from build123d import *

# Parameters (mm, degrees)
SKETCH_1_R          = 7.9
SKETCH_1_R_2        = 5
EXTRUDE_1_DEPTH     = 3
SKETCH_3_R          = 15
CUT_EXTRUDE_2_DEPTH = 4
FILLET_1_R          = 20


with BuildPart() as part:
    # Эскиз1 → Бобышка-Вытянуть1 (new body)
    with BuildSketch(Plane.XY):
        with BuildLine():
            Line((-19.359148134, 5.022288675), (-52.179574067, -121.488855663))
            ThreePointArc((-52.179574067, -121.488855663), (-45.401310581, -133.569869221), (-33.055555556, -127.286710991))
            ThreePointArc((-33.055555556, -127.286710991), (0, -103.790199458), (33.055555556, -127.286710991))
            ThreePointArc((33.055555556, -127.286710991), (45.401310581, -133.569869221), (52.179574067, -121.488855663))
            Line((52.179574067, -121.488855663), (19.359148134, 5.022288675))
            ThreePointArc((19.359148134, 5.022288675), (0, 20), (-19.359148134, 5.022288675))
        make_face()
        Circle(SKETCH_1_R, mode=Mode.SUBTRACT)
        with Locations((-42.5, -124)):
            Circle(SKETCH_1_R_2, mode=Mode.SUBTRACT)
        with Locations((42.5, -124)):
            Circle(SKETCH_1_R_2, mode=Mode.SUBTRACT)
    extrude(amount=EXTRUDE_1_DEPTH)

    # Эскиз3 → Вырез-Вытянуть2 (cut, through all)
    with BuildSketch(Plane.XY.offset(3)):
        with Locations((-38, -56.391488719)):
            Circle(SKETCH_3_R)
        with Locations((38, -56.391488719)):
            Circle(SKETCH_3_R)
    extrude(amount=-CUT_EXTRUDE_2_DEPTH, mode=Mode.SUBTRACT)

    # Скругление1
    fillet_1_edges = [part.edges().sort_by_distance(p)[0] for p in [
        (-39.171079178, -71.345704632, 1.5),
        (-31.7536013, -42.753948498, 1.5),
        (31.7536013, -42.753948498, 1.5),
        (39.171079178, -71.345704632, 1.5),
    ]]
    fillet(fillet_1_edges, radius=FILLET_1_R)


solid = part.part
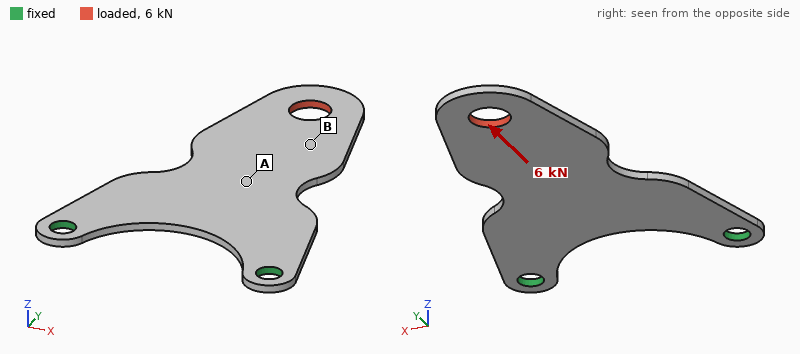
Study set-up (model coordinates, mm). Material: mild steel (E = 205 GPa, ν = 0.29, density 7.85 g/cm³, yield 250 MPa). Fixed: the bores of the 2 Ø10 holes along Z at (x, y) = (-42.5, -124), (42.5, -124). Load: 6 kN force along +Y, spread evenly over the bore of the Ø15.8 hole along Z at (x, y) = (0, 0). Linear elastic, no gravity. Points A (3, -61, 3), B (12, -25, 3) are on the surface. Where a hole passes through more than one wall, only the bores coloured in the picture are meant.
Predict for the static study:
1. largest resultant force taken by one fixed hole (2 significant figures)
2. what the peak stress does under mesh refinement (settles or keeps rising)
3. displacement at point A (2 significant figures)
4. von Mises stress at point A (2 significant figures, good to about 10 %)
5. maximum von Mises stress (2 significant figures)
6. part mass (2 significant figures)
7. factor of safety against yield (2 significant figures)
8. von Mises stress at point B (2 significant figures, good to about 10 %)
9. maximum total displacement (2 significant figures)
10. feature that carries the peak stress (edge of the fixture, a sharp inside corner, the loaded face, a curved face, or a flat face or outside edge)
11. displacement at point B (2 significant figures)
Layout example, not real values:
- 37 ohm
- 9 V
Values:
- 3.3 kN
- settles
- 15 µm
- 27 MPa
- 120 MPa
- 190 g
- 2.1
- 43 MPa
- 34 µm
- the loaded face
- 22 µm
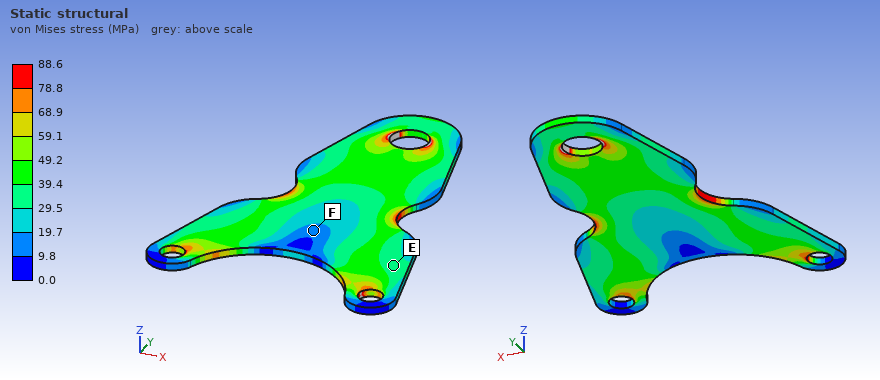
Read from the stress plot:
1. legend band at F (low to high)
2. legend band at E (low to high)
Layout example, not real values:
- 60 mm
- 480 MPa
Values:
- 9.8 to 19.7 MPa
- 29.5 to 39.4 MPa
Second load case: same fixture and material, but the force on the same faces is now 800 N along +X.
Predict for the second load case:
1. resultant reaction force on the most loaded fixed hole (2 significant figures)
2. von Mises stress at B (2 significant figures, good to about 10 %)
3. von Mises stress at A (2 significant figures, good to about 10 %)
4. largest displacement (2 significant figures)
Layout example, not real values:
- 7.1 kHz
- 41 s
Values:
- 1.2 kN
- 10 MPa
- 6.5 MPa
- 47 µm
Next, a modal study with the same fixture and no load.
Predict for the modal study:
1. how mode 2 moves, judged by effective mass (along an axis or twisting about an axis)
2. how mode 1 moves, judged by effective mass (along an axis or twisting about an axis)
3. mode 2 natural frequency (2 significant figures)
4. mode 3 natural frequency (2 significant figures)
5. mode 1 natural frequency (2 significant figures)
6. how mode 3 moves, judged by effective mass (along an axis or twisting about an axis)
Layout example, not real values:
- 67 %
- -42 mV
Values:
- along Z
- along Z
- 780 Hz
- 900 Hz
- 150 Hz
- twisting about Y
